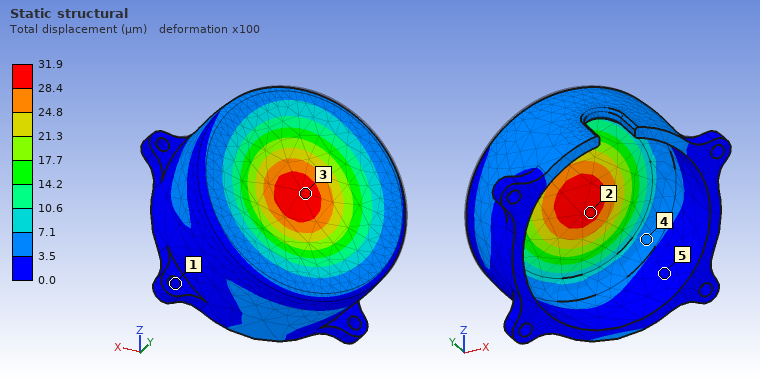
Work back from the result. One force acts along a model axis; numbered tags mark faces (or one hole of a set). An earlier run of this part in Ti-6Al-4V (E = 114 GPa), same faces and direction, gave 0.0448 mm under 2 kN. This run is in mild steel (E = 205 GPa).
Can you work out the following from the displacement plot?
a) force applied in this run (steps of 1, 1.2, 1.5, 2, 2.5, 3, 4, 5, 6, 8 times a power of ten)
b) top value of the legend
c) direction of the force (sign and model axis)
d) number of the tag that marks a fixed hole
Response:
2.5 kN
31.9 µm
-Y
1
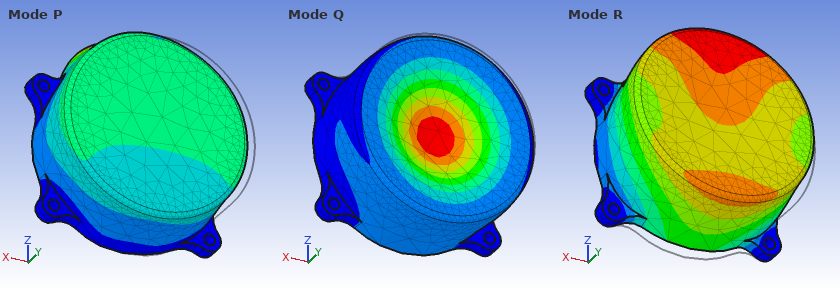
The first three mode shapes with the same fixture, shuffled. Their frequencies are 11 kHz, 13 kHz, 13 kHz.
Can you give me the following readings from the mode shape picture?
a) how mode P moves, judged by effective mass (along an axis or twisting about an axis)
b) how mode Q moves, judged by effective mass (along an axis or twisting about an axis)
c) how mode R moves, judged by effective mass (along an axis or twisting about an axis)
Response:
along X
along Y
along Z
